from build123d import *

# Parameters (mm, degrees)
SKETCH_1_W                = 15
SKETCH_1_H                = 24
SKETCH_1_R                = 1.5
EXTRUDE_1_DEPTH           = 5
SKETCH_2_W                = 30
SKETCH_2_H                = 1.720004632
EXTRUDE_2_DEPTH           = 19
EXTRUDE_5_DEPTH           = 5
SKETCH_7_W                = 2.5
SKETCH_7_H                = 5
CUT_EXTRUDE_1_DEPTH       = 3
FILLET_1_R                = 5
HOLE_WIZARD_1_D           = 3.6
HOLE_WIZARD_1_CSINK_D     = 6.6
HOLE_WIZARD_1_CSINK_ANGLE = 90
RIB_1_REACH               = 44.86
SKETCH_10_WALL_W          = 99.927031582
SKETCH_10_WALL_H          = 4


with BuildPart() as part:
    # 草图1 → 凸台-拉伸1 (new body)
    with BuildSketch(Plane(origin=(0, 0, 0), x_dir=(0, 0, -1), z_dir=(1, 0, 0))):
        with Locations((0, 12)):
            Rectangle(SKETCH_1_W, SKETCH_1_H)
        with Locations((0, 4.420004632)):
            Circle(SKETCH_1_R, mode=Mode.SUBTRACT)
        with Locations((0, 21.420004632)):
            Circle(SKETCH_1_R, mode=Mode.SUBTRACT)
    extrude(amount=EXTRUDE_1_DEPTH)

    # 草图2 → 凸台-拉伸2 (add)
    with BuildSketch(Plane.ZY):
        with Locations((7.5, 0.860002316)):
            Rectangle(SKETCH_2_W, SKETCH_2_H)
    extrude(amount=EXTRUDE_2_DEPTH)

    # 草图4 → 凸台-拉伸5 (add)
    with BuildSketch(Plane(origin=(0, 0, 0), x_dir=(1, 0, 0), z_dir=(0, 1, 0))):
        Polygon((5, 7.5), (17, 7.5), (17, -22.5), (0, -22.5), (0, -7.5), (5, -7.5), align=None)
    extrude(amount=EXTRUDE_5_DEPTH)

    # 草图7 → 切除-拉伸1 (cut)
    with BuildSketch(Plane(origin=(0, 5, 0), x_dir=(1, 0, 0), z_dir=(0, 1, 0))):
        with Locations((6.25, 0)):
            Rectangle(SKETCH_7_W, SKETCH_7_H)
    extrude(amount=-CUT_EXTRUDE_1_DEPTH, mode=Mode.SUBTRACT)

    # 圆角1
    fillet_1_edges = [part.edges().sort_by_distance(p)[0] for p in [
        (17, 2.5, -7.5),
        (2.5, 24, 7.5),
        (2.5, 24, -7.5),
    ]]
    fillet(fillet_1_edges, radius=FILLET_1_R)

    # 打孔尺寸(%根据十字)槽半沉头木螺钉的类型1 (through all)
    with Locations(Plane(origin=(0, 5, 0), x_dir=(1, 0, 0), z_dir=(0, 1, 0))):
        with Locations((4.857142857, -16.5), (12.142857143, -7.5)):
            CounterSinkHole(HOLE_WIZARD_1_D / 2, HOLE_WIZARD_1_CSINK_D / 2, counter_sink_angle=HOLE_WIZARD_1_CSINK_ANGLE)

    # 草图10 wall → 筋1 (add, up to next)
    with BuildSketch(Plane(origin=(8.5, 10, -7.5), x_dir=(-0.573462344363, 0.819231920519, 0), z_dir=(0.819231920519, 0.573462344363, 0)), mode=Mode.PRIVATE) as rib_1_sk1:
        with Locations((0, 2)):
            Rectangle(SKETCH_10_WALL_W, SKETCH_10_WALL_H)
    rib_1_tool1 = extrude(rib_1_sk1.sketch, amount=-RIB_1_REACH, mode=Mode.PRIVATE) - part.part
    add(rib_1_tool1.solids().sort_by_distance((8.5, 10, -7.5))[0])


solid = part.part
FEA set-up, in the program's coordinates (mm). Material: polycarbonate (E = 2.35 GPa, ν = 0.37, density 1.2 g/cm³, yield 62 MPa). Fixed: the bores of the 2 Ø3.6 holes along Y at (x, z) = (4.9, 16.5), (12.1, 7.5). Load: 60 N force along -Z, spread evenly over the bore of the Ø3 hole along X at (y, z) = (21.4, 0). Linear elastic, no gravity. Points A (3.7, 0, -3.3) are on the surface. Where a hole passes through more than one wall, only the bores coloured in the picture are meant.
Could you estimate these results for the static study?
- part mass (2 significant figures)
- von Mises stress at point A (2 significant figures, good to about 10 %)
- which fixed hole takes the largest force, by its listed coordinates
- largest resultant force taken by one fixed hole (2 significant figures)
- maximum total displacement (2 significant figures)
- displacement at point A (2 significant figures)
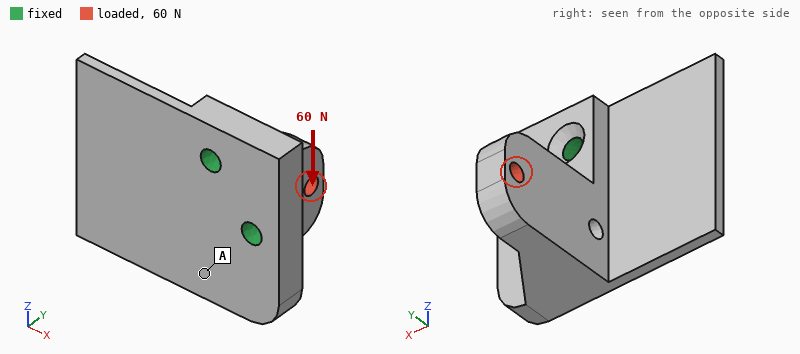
5.7 g
2.9 MPa
(4.9, 16.5)
82 N
0.59 mm
0.22 mm
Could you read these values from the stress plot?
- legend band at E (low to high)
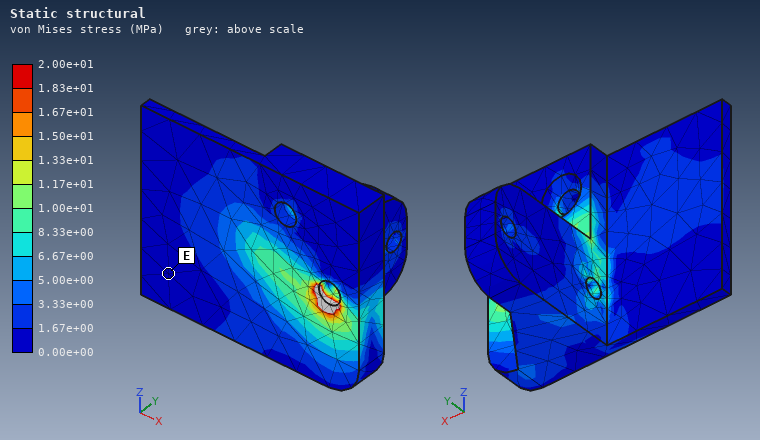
0.00e+00 to 1.67e+00 MPa
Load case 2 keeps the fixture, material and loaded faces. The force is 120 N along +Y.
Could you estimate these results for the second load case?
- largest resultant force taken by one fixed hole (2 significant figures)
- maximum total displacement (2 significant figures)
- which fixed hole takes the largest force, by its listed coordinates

100 N
0.63 mm
(12.1, 7.5)
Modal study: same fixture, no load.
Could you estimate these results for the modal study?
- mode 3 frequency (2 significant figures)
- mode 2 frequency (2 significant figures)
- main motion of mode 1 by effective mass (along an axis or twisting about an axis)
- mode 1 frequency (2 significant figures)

1900 Hz
1400 Hz
along Y
940 Hz
